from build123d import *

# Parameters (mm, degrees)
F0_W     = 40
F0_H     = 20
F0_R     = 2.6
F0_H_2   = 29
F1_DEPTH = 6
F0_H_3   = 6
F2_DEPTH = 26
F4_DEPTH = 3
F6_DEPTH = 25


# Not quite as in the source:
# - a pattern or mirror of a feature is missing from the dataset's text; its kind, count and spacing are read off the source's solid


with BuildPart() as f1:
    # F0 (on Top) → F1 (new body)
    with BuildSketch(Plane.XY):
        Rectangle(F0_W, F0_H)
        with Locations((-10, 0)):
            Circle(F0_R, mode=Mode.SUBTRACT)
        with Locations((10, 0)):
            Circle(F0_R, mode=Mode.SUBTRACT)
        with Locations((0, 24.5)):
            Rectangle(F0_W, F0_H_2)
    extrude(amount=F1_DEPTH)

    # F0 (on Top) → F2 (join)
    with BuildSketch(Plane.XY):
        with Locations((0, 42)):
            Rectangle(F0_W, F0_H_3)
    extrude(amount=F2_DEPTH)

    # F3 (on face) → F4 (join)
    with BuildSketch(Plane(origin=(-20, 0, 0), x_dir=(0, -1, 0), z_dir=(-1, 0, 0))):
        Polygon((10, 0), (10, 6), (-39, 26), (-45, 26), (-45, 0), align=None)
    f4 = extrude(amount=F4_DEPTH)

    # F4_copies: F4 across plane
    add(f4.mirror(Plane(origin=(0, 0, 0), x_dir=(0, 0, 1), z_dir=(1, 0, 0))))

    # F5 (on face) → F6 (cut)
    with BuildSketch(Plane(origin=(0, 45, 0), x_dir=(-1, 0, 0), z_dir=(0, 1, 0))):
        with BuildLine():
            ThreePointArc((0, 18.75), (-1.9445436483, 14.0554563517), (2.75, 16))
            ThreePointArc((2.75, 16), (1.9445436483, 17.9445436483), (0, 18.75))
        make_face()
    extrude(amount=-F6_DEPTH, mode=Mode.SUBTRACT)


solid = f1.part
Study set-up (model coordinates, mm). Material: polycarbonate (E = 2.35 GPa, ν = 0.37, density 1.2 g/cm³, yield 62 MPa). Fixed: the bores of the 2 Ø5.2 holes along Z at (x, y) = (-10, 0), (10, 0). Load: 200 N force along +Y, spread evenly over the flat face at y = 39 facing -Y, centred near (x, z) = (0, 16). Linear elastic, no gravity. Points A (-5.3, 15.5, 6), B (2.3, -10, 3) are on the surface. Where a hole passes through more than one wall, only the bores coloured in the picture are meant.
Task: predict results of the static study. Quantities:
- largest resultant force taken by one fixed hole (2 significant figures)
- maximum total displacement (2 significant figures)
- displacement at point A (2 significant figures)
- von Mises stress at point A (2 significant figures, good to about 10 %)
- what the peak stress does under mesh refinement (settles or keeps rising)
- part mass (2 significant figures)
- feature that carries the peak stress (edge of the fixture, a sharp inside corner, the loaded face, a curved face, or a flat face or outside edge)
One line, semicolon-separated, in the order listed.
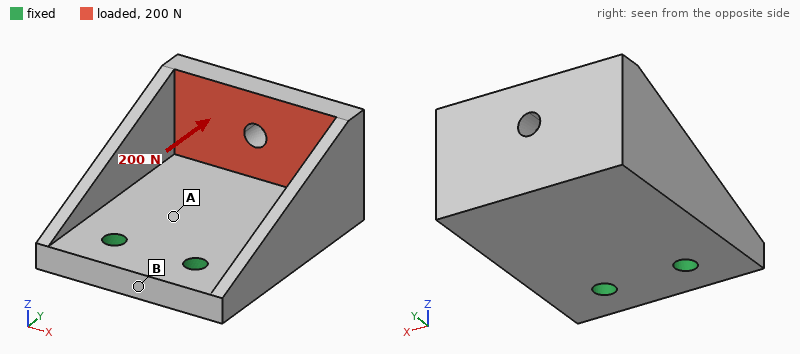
100 N; 0.73 mm; 0.11 mm; 3.6 MPa; keeps rising; 28 g; edge of the fixture
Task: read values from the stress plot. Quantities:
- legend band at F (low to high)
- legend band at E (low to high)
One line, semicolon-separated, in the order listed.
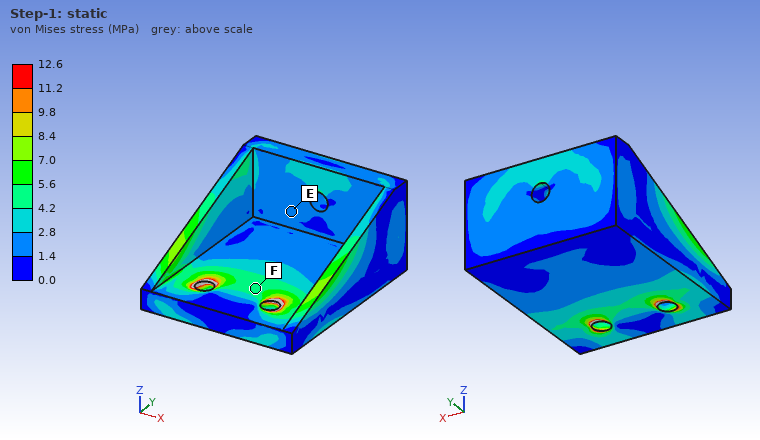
4.2 to 5.6 MPa; 1.4 to 2.8 MPa
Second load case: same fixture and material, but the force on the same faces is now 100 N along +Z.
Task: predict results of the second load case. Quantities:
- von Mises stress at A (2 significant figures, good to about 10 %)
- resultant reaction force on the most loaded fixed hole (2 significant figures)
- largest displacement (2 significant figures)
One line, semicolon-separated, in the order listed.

3.7 MPa; 50 N; 0.81 mm
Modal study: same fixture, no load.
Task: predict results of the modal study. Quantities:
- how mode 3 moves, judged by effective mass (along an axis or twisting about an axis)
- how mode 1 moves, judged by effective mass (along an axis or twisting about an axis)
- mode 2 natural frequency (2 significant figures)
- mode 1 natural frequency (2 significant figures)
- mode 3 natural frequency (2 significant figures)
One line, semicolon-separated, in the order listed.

along X; along Z; 840 Hz; 510 Hz; 1800 Hz
